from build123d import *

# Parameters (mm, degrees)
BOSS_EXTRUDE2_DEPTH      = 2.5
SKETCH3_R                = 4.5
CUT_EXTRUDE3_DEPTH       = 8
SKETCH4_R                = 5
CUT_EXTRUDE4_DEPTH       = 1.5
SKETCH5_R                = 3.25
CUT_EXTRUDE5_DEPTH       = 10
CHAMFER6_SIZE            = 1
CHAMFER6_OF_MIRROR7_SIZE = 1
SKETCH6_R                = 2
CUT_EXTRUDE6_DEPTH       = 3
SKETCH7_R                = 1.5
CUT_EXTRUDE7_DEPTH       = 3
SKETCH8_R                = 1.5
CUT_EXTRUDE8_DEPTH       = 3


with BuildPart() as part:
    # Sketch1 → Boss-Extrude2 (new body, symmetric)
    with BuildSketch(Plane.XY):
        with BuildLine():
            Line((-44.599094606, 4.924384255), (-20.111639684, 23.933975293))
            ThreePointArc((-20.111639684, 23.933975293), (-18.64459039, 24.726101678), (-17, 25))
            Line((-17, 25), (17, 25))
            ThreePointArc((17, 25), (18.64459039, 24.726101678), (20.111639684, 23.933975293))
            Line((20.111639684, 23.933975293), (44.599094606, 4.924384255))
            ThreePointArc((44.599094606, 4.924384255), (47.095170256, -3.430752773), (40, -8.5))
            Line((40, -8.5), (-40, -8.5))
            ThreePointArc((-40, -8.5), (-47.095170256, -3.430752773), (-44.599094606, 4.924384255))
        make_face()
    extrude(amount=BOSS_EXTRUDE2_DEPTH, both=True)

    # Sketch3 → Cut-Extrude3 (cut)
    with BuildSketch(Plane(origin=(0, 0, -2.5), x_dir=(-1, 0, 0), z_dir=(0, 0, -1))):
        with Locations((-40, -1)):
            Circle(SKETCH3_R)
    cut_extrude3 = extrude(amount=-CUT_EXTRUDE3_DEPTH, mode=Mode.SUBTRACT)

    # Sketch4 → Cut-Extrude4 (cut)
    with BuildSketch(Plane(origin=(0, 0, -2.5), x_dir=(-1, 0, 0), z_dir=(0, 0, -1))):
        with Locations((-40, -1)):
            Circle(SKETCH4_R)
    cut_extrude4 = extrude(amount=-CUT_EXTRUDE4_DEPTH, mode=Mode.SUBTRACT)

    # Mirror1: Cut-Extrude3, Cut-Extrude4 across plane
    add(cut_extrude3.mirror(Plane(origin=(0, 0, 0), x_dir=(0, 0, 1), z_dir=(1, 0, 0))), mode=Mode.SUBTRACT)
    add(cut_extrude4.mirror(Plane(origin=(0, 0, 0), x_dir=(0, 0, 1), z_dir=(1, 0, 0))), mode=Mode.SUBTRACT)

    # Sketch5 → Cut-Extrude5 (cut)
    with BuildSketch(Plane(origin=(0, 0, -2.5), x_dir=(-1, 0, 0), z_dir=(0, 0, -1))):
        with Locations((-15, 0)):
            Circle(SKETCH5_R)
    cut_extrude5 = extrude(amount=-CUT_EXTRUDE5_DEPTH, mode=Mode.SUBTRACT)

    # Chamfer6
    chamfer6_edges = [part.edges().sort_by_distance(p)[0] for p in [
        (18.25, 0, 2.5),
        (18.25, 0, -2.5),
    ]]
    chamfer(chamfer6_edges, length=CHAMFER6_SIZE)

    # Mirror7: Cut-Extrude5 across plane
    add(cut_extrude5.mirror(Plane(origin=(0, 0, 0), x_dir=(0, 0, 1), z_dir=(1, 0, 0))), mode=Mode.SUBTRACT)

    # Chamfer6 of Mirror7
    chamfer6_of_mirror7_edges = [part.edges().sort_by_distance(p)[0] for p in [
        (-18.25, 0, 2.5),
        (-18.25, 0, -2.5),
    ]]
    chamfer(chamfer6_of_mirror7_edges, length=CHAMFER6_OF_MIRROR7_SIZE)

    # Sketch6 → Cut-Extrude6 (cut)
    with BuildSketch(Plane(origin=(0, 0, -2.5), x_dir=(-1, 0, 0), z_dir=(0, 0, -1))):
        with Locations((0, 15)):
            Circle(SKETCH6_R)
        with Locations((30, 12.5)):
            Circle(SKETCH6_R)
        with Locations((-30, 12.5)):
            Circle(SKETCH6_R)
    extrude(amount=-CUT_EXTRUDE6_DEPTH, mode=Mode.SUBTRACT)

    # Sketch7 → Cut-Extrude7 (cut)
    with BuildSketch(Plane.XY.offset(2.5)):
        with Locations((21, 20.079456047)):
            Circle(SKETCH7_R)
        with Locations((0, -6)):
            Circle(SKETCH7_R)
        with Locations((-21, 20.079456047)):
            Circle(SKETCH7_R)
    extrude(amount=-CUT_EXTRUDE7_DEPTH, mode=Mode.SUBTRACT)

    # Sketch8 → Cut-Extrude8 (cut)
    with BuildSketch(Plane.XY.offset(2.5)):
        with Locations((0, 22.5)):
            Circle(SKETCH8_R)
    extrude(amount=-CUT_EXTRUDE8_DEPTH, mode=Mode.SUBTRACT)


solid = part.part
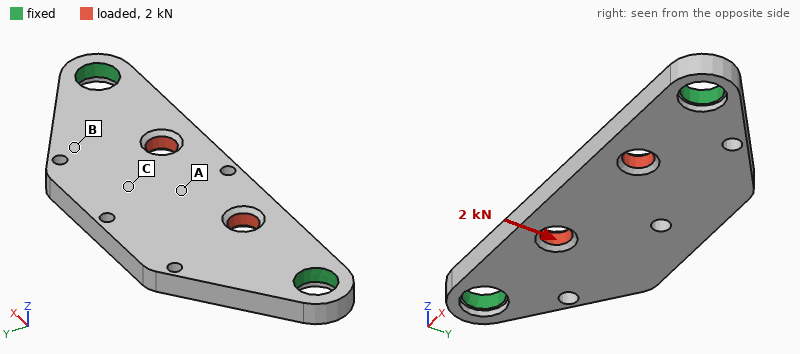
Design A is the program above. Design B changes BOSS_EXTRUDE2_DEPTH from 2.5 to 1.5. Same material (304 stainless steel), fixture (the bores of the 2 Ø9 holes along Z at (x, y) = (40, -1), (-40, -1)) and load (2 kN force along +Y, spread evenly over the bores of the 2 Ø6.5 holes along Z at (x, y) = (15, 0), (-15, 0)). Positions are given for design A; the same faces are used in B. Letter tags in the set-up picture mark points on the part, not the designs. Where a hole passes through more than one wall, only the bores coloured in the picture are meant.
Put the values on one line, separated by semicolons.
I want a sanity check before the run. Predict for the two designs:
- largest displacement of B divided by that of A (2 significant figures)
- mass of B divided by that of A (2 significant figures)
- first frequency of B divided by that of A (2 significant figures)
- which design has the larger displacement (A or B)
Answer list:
1.6; 0.60; 0.66; B
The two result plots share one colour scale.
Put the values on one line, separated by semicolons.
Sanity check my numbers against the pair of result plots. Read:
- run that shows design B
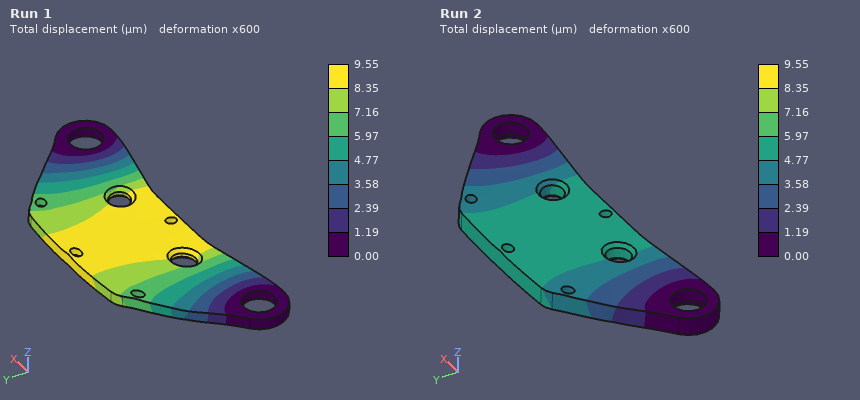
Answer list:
Run 1
